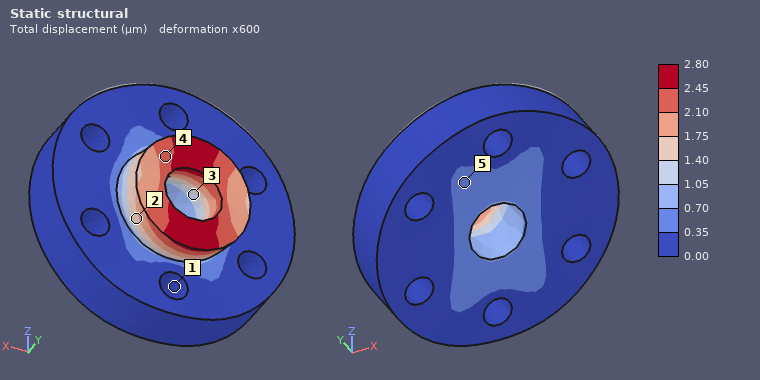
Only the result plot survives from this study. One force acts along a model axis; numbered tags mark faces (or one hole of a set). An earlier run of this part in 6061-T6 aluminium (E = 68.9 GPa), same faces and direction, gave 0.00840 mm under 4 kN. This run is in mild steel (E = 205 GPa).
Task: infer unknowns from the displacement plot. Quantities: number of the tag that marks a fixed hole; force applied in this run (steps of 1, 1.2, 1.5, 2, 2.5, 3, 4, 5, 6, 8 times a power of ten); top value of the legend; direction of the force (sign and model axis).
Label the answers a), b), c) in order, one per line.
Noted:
a) 1
b) 4 kN
c) 2.80 µm
d) -Z
